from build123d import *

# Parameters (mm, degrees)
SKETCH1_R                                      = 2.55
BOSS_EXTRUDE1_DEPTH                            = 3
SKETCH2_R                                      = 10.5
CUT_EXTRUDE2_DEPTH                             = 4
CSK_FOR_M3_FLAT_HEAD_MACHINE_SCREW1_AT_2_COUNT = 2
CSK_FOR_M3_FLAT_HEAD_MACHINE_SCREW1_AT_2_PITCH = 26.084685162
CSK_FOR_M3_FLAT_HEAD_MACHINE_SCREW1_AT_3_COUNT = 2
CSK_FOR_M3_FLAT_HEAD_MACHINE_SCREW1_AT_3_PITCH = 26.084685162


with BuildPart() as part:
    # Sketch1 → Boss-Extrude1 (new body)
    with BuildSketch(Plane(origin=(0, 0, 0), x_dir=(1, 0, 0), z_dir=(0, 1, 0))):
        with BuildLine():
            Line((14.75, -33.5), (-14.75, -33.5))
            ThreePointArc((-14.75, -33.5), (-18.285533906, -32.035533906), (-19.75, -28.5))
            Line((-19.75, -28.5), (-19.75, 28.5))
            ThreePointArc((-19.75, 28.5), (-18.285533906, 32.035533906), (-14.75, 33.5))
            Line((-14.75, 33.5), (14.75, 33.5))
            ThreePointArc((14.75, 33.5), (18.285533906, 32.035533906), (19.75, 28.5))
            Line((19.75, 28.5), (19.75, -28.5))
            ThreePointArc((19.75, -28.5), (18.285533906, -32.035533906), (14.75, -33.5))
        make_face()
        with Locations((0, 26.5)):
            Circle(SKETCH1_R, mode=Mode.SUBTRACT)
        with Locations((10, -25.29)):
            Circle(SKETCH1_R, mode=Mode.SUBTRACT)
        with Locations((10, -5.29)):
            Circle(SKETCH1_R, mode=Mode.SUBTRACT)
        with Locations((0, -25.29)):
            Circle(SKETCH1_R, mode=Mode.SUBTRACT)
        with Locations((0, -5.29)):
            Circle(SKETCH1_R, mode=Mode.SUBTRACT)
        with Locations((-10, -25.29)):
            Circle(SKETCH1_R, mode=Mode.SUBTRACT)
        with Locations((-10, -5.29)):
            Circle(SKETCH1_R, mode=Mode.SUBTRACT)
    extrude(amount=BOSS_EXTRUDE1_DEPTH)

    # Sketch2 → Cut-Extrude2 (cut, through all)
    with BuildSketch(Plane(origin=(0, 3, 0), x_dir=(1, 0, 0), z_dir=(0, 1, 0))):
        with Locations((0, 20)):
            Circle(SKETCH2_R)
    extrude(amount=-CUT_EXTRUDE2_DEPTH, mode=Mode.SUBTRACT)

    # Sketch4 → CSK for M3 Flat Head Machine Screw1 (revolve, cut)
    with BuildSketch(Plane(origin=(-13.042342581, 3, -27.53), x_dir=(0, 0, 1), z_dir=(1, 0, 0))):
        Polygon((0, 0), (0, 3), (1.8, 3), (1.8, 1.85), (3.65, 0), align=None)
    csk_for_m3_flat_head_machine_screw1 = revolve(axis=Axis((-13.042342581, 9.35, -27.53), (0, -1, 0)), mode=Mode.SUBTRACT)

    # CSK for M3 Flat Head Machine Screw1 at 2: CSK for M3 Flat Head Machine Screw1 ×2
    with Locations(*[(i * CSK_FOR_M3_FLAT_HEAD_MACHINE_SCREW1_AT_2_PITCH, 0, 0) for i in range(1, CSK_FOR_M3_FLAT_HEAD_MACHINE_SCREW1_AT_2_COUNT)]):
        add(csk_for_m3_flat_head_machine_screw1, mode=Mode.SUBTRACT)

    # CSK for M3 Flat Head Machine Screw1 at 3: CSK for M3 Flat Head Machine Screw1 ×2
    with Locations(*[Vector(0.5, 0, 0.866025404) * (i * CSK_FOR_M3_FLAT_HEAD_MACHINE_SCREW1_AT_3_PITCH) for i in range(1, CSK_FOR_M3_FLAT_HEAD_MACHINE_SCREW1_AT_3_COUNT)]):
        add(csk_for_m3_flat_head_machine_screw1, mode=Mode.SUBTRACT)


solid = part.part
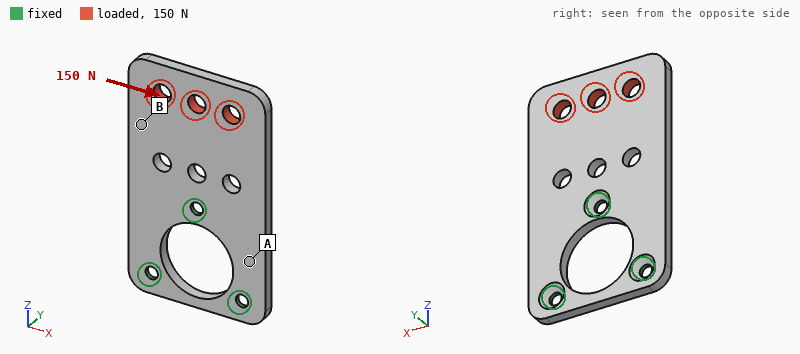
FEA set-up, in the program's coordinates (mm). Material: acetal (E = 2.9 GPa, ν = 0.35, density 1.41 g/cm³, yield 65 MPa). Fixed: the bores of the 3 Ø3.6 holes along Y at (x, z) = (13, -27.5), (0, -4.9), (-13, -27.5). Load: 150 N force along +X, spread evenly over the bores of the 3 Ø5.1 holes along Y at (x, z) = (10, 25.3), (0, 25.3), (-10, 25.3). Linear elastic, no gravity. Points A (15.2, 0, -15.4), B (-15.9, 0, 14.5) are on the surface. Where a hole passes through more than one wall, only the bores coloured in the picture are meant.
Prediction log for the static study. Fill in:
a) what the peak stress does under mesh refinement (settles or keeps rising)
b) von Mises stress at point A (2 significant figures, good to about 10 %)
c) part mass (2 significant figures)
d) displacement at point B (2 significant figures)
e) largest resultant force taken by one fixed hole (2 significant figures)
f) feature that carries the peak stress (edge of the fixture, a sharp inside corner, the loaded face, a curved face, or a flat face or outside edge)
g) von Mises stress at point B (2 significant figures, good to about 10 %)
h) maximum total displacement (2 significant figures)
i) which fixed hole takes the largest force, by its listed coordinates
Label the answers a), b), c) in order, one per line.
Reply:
a) keeps rising
b) 5.9 MPa
c) 8.9 g
d) 0.14 mm
e) 190 N
f) edge of the fixture
g) 1.9 MPa
h) 0.25 mm
i) (0, -4.9)
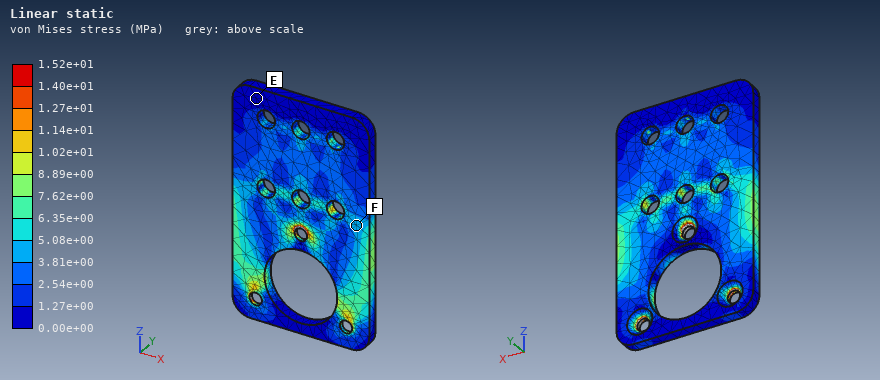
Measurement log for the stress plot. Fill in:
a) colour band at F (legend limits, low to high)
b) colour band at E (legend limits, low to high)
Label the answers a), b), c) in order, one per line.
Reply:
a) 3.81e+00 to 5.08e+00 MPa
b) 0.00e+00 to 1.27e+00 MPa
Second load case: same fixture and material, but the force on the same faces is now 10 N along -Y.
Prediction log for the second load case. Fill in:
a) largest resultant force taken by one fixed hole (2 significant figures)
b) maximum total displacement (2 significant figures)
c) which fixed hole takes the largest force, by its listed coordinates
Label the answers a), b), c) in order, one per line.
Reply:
a) 30 N
b) 0.83 mm
c) (0, -4.9)
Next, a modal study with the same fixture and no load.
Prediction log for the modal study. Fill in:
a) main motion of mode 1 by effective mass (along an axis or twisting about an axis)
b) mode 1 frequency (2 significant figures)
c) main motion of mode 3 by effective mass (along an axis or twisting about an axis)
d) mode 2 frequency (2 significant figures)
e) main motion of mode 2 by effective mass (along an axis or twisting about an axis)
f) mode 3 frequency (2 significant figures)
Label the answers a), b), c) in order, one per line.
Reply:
a) along Y
b) 380 Hz
c) along Y
d) 650 Hz
e) twisting about Z
f) 1700 Hz
